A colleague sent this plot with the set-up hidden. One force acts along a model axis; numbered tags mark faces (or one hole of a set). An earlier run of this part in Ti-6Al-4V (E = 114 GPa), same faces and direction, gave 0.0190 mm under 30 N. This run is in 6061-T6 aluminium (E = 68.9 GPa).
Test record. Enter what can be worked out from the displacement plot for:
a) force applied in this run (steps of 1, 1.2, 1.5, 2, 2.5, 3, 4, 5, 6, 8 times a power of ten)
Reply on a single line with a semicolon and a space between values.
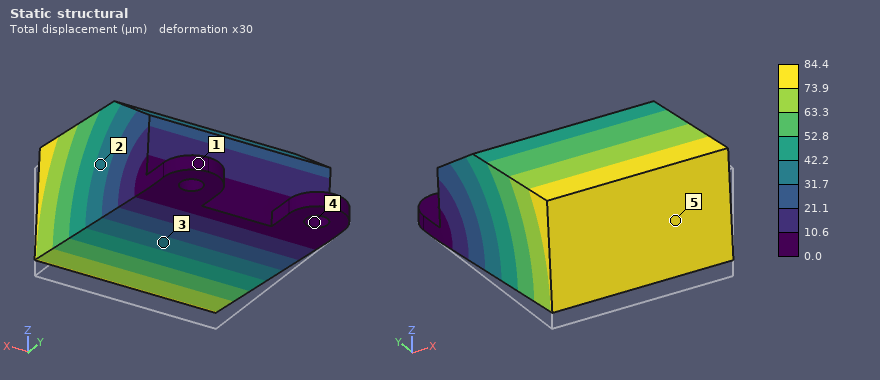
80 N
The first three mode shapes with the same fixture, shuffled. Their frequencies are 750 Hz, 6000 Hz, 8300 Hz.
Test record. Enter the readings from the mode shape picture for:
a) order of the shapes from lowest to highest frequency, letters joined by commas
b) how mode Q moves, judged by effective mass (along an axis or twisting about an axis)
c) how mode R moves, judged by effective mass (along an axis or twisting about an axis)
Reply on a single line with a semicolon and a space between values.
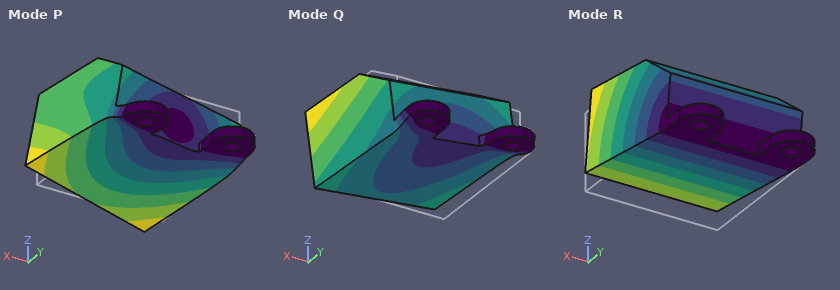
R, Q, P; along X; along Z
